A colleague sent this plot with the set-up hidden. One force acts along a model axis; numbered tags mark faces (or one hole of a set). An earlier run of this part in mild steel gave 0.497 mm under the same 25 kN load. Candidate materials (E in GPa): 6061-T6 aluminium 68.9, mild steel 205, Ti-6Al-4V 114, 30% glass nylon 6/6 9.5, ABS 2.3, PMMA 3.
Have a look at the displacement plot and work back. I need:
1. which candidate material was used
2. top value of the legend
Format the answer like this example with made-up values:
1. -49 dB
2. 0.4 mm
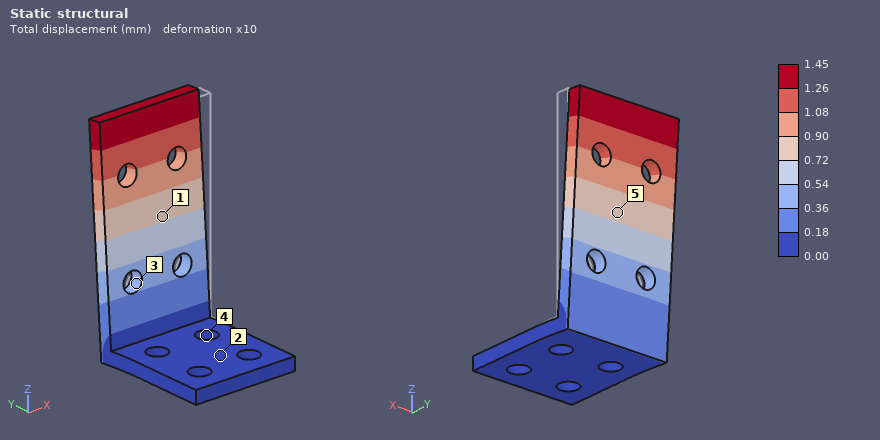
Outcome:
1. 6061-T6 aluminium
2. 1.45 mm
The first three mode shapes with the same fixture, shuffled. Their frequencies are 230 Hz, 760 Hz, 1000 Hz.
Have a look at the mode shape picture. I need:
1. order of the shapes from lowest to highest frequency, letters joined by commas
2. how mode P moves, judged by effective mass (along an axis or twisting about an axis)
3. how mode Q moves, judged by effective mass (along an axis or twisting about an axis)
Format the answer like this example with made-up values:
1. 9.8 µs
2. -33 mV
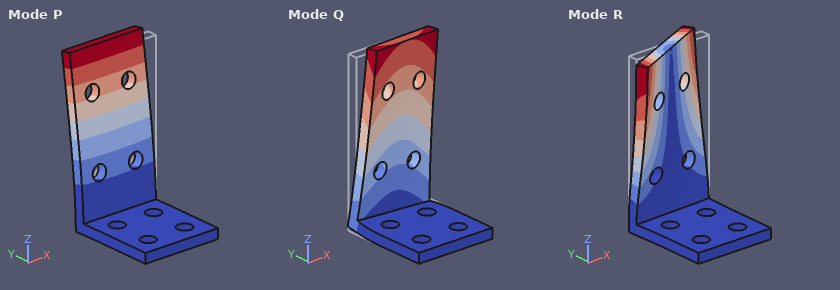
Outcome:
1. P, Q, R
2. along Y
3. along X
